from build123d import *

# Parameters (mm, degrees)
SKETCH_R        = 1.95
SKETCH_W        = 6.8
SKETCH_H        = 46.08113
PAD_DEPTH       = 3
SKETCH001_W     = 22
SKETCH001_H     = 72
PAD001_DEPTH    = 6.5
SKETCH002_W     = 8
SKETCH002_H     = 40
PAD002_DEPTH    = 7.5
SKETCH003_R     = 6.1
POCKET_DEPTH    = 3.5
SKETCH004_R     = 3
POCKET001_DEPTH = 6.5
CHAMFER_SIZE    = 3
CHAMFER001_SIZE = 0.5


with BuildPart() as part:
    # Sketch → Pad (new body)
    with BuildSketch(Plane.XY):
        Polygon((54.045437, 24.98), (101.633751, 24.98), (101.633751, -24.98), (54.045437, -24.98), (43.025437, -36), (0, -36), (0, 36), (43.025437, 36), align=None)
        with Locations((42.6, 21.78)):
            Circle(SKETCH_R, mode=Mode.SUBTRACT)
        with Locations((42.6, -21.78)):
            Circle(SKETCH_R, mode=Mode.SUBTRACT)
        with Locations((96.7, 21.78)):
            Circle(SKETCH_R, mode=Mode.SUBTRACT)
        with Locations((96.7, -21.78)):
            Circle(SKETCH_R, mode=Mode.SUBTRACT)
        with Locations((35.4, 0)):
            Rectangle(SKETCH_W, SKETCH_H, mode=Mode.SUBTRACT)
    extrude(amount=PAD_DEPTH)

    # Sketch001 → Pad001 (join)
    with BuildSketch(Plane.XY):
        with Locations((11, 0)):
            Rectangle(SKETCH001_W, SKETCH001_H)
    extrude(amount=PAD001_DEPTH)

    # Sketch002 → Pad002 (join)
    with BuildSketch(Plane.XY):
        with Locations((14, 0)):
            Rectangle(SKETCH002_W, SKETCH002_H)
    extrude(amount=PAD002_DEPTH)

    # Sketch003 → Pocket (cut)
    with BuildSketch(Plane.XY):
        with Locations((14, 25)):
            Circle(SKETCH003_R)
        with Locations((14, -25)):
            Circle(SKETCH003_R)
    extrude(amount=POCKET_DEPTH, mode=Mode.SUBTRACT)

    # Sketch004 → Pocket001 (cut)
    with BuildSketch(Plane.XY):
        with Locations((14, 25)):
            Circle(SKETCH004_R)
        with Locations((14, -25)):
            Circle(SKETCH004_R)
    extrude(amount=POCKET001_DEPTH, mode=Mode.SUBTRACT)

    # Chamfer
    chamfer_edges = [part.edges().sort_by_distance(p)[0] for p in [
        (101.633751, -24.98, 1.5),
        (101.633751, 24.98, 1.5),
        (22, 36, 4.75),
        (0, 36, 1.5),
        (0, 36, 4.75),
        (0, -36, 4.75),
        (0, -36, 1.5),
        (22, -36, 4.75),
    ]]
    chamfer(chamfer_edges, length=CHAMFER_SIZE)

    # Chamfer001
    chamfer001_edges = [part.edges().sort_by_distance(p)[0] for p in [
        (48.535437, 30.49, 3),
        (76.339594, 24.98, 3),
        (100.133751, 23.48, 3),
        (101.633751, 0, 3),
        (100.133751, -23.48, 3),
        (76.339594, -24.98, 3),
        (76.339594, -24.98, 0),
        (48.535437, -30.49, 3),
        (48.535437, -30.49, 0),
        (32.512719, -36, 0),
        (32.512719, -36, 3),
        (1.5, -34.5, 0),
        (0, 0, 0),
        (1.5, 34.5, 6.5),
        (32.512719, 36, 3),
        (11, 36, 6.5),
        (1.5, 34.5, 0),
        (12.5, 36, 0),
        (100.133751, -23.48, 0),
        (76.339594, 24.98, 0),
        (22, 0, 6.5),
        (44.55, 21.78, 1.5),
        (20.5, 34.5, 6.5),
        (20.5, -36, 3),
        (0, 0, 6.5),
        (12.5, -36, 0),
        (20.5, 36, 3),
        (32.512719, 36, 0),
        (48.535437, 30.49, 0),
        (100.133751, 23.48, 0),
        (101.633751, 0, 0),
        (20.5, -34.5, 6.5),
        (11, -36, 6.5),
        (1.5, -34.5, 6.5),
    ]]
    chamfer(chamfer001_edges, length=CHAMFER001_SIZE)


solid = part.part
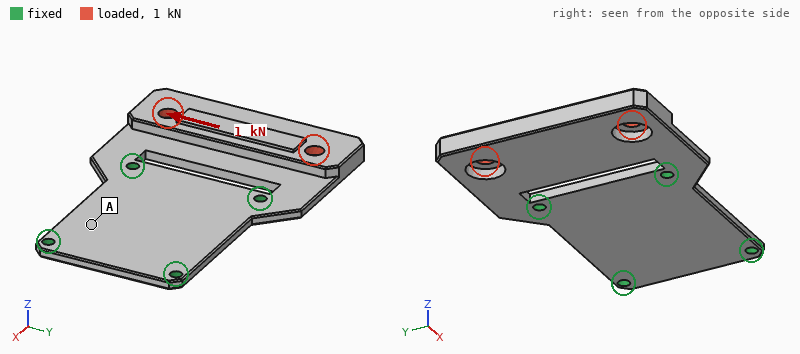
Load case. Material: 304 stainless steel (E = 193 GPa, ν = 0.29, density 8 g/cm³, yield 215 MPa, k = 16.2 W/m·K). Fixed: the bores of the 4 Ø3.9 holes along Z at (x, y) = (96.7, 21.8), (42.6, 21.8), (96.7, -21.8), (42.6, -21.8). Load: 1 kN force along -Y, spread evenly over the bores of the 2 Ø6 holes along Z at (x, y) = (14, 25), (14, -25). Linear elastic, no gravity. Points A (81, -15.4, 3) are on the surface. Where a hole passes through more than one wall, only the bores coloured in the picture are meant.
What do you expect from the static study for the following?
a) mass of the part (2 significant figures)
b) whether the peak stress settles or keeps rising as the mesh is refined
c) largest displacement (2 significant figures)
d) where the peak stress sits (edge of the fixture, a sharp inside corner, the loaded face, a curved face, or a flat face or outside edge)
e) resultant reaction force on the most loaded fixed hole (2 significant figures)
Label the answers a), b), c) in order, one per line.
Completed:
a) 180 g
b) keeps rising
c) 25 µm
d) edge of the fixture
e) 710 N
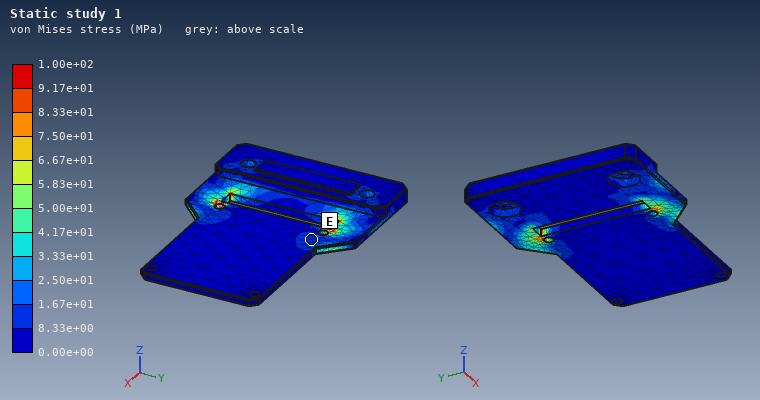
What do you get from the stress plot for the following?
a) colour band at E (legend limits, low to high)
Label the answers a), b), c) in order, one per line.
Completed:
a) 8.33e+00 to 1.67e+01 MPa
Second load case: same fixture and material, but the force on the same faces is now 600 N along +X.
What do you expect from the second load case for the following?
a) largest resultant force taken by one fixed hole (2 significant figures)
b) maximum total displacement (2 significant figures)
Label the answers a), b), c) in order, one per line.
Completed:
a) 290 N
b) 0.13 mm
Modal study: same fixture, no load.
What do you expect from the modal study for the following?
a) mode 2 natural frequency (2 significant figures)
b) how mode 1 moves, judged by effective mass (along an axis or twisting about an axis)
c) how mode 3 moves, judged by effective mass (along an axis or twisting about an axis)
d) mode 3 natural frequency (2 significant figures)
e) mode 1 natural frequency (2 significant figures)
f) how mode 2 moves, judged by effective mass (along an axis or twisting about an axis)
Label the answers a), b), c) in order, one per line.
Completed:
a) 2100 Hz
b) along Z
c) along Z
d) 4100 Hz
e) 540 Hz
f) twisting about X
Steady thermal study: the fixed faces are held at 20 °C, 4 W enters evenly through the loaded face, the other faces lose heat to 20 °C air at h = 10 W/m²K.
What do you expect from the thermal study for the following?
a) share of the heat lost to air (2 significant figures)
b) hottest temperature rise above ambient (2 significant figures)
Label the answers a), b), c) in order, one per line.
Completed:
a) 55 %
b) 45 K
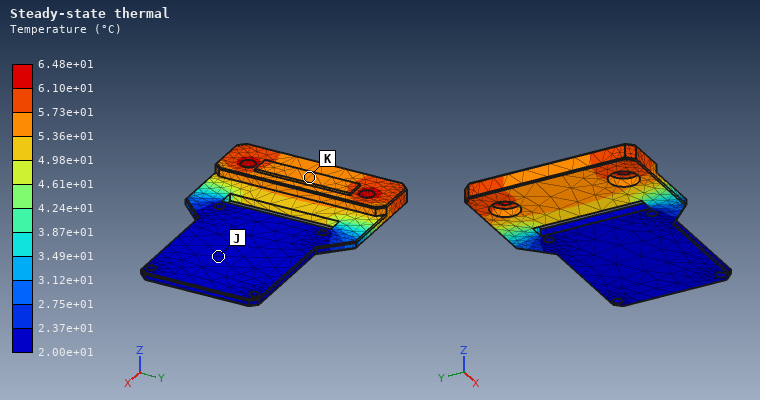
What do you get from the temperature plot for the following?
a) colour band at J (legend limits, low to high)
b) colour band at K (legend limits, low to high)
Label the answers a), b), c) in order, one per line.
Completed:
a) 2.00e+01 to 2.37e+01 °C
b) 5.36e+01 to 5.73e+01 °C
